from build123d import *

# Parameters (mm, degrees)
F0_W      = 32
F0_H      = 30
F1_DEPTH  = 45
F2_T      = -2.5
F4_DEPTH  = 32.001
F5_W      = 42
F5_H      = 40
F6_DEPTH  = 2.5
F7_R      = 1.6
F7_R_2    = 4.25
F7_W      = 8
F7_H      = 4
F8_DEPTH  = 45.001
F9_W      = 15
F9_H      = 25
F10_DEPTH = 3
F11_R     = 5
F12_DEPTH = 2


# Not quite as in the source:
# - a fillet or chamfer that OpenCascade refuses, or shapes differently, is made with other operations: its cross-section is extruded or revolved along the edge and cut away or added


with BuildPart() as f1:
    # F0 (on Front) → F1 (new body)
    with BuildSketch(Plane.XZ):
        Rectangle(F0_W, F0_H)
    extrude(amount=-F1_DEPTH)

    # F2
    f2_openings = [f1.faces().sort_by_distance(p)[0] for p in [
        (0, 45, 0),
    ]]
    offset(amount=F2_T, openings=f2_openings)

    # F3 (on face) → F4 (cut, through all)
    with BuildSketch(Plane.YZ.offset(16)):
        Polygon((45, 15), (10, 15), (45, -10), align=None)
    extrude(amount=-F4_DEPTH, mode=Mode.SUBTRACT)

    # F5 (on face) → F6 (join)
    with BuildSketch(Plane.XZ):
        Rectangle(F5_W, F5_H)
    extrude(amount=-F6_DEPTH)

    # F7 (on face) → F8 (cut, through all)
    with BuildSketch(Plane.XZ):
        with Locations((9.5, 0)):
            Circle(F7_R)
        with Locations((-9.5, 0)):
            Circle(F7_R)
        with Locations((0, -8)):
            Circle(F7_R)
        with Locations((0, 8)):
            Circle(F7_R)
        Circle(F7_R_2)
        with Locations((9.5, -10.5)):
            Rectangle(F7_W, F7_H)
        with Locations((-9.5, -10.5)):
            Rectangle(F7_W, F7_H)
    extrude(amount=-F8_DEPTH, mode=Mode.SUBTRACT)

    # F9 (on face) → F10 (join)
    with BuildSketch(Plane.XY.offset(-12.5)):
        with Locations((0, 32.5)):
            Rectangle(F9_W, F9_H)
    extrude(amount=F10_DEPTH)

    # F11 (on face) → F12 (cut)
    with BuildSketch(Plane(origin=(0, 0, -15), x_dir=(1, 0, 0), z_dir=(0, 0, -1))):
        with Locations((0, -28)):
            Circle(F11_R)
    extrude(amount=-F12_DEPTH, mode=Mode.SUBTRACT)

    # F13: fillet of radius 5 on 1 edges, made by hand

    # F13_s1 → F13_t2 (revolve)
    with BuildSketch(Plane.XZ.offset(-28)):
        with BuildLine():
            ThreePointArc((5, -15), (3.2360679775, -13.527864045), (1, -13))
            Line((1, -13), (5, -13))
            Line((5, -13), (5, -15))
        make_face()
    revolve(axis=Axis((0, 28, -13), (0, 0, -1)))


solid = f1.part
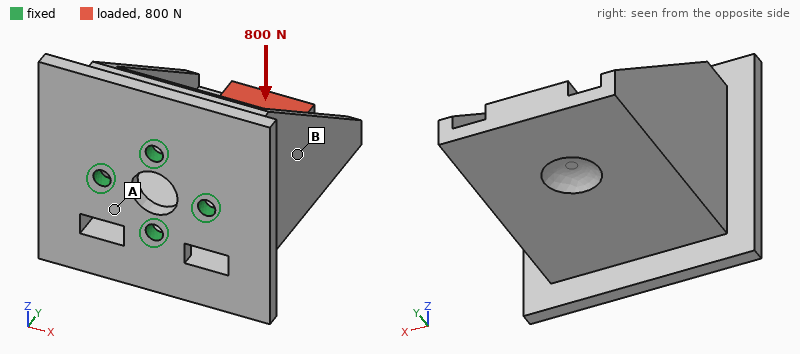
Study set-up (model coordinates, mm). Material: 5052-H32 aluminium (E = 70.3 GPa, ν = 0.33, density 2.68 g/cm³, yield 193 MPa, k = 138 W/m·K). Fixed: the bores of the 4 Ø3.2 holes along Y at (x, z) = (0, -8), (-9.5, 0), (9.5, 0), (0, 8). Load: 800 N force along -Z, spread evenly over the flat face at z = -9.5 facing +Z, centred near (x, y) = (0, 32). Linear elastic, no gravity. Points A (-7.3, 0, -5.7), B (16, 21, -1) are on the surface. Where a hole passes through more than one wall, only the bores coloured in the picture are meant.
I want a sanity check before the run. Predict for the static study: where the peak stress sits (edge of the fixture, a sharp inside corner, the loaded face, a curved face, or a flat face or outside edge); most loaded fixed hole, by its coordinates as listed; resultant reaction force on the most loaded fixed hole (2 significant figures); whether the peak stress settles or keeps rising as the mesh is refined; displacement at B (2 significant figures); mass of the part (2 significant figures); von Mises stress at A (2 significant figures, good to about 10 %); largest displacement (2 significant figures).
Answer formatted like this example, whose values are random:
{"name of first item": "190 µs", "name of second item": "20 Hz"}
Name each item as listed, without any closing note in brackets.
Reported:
{"where the peak stress sits": "edge of the fixture", "most loaded fixed hole, by its coordinates as listed": "(0, -8)", "resultant reaction force on the most loaded fixed hole": "1.0 kN", "whether the peak stress settles or keeps rising as the mesh is refined": "keeps rising", "displacement at B": "0.067 mm", "mass of the part": "34 g", "von Mises stress at A": "30 MPa", "largest displacement": "0.20 mm"}
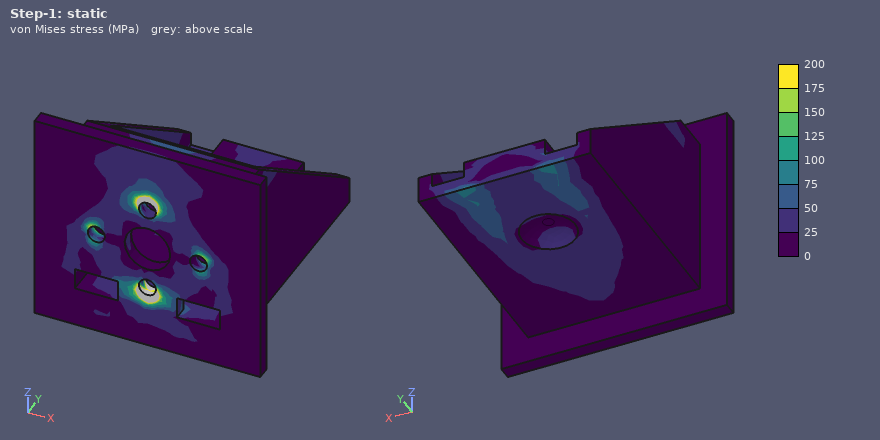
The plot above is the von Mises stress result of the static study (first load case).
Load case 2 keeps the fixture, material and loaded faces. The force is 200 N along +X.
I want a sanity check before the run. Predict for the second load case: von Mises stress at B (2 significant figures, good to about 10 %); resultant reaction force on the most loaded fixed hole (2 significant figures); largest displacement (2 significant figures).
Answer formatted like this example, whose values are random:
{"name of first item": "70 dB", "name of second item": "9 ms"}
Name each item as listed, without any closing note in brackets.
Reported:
{"von Mises stress at B": "13 MPa", "resultant reaction force on the most loaded fixed hole": "230 N", "largest displacement": "83 µm"}
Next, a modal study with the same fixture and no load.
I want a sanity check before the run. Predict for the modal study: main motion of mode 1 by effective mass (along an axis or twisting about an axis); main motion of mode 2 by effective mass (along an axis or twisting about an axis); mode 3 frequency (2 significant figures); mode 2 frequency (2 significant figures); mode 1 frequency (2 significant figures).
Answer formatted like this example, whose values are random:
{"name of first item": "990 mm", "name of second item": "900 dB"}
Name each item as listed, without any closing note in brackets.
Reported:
{"main motion of mode 1 by effective mass": "along X", "main motion of mode 2 by effective mass": "along Z", "mode 3 frequency": "6500 Hz", "mode 2 frequency": "3300 Hz", "mode 1 frequency": "2700 Hz"}
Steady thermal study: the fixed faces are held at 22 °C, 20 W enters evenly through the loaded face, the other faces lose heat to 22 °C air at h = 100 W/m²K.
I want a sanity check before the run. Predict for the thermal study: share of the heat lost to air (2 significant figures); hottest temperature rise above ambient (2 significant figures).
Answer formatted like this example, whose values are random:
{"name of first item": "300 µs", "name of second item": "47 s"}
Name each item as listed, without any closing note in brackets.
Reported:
{"share of the heat lost to air": "44 %", "hottest temperature rise above ambient": "28 K"}
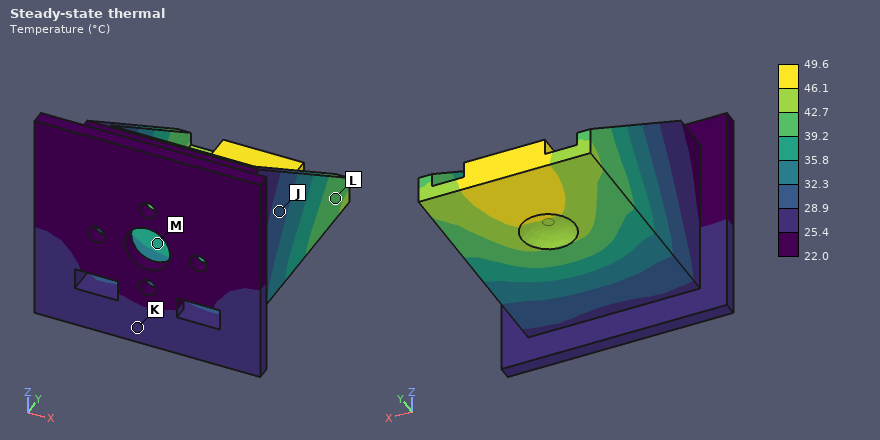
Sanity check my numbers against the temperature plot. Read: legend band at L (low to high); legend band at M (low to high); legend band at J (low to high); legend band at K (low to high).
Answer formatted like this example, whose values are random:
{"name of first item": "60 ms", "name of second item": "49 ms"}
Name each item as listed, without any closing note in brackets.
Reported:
{"legend band at L": "39.2 to 42.7 °C", "legend band at M": "35.8 to 39.2 °C", "legend band at J": "28.9 to 32.3 °C", "legend band at K": "25.4 to 28.9 °C"}
